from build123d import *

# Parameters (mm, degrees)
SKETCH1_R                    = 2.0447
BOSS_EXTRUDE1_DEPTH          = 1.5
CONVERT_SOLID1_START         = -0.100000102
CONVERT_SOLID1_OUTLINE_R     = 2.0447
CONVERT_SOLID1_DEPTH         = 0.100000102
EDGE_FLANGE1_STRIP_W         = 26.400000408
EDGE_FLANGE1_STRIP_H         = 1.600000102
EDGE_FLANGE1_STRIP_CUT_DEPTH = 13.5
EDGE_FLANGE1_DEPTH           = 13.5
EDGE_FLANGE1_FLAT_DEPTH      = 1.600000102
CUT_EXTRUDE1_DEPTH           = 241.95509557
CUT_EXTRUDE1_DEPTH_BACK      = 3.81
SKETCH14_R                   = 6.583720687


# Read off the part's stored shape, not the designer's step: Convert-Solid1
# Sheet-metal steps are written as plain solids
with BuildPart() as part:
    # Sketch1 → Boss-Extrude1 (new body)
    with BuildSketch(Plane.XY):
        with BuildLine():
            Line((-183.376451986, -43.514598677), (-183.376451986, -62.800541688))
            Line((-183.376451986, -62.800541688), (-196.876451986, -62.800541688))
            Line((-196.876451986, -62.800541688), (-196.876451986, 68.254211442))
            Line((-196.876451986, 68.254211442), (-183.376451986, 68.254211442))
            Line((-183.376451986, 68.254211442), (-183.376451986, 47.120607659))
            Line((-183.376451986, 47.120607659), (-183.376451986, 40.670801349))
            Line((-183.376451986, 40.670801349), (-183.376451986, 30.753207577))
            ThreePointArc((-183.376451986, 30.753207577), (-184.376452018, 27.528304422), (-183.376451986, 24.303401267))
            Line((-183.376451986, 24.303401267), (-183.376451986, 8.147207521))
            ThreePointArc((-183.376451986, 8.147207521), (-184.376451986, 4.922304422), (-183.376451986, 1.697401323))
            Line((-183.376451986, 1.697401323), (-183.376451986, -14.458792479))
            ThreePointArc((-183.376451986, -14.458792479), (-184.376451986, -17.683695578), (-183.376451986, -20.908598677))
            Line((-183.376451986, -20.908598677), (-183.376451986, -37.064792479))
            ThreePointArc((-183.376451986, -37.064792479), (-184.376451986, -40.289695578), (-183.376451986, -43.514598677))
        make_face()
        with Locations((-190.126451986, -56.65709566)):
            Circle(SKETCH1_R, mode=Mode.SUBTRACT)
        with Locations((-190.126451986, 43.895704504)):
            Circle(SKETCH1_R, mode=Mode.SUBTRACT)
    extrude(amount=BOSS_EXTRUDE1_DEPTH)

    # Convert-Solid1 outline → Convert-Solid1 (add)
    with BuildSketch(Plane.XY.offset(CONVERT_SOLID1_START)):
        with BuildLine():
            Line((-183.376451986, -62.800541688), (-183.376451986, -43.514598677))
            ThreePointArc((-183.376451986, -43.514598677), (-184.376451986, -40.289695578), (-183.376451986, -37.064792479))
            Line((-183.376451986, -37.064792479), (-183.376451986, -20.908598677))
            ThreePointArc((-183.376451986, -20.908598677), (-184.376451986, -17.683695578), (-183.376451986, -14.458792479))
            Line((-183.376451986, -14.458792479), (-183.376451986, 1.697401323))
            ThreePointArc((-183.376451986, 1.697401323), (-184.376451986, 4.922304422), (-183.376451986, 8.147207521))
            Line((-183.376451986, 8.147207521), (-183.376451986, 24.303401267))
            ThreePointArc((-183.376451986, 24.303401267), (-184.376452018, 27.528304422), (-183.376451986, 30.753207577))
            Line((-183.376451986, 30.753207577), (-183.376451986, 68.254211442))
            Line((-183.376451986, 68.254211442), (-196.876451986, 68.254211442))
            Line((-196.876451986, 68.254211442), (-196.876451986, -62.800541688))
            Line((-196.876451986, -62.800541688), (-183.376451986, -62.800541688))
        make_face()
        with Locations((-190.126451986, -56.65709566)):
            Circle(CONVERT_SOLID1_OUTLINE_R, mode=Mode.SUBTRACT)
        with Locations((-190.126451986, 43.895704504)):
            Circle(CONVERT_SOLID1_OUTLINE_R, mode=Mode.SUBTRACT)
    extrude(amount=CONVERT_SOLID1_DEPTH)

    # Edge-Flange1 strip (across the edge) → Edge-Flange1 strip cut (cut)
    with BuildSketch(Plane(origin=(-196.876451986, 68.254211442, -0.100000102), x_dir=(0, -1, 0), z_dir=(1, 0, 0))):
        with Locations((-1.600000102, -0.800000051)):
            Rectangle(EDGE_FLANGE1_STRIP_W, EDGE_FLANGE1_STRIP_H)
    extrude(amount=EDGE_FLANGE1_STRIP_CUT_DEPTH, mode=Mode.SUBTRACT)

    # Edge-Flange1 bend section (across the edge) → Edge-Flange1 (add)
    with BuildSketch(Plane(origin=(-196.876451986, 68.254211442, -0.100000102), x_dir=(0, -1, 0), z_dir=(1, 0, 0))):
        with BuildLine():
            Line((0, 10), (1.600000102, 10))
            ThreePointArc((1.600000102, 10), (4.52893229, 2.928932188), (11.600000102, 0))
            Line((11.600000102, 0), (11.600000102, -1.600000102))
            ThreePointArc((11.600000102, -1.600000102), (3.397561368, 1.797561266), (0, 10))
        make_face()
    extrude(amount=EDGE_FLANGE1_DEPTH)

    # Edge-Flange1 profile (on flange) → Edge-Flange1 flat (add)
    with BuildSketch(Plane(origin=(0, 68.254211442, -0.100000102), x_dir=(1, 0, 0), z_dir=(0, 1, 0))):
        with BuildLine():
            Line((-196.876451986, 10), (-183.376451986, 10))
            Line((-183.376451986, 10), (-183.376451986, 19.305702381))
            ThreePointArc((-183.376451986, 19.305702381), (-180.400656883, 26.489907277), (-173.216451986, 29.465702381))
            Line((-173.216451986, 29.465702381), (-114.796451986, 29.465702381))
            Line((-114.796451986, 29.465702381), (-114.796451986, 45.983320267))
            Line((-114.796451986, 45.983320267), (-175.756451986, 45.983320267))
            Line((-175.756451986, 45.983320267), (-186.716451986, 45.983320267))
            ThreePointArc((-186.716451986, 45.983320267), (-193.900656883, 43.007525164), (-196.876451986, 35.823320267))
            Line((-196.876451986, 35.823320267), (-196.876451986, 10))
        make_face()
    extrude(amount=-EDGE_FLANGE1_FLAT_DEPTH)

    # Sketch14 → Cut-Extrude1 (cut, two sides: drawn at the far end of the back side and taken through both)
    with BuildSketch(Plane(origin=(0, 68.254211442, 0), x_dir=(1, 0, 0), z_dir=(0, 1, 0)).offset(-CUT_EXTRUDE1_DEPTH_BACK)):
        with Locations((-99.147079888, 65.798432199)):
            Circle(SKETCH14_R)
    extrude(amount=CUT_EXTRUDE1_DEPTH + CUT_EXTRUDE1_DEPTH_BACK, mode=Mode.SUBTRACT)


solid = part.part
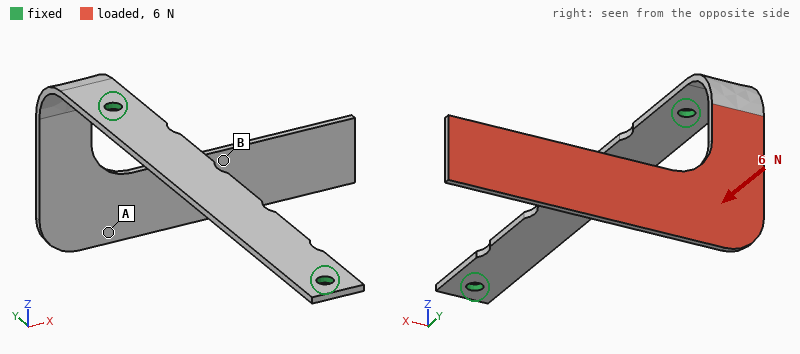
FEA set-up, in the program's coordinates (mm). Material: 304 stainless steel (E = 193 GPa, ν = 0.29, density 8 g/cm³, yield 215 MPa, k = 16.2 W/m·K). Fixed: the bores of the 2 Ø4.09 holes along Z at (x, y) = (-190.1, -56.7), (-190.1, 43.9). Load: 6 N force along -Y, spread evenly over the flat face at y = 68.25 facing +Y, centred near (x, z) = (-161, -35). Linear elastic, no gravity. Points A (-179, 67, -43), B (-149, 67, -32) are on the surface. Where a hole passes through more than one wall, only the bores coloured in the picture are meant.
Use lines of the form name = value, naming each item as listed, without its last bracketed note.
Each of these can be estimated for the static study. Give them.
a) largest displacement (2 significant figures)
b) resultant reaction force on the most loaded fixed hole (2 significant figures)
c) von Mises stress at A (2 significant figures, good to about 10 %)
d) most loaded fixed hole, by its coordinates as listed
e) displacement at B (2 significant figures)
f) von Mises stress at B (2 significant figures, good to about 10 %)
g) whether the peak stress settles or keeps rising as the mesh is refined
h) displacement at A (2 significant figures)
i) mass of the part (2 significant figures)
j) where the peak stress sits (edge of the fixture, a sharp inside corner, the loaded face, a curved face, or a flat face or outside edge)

largest displacement = 0.80 mm
resultant reaction force on the most loaded fixed hole = 6.0 N
von Mises stress at A = 14 MPa
most loaded fixed hole, by its coordinates as listed = (-190.1, 43.9)
displacement at B = 0.44 mm
von Mises stress at B = 5.2 MPa
whether the peak stress settles or keeps rising as the mesh is refined = keeps rising
displacement at A = 0.35 mm
mass of the part = 44 g
where the peak stress sits = edge of the fixture
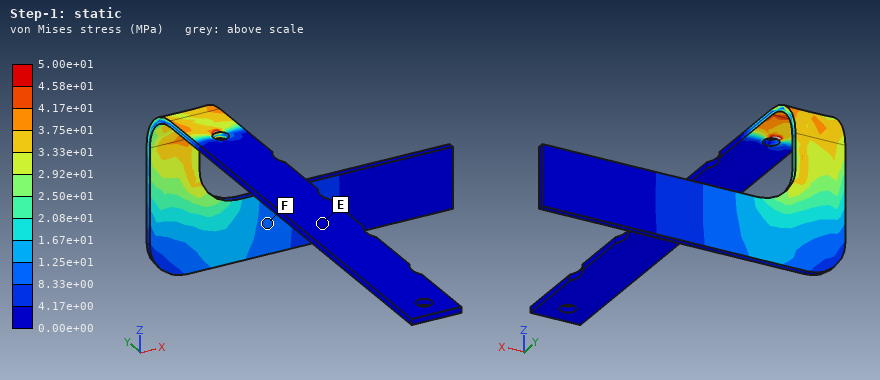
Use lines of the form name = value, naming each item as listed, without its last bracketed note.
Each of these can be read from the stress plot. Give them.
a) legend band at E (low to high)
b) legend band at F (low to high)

legend band at E = 0.00e+00 to 4.17e+00 MPa
legend band at F = 8.33e+00 to 1.25e+01 MPa
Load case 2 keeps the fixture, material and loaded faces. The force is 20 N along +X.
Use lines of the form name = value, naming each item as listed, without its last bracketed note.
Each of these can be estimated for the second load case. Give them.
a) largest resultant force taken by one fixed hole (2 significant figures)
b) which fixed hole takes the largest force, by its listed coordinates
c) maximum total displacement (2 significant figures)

largest resultant force taken by one fixed hole = 21 N
which fixed hole takes the largest force, by its listed coordinates = (-190.1, 43.9)
maximum total displacement = 0.85 mm
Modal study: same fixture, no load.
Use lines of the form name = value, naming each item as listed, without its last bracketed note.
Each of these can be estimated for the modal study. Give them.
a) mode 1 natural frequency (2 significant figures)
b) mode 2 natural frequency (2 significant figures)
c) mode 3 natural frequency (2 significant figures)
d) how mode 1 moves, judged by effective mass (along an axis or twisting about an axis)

mode 1 natural frequency = 120 Hz
mode 2 natural frequency = 180 Hz
mode 3 natural frequency = 320 Hz
how mode 1 moves, judged by effective mass = along Y
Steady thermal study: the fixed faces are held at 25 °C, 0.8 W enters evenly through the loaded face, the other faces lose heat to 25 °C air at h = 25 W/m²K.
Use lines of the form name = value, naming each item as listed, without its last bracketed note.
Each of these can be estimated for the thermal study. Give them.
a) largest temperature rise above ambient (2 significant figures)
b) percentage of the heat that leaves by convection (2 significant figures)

largest temperature rise above ambient = 15 K
percentage of the heat that leaves by convection = 93 %
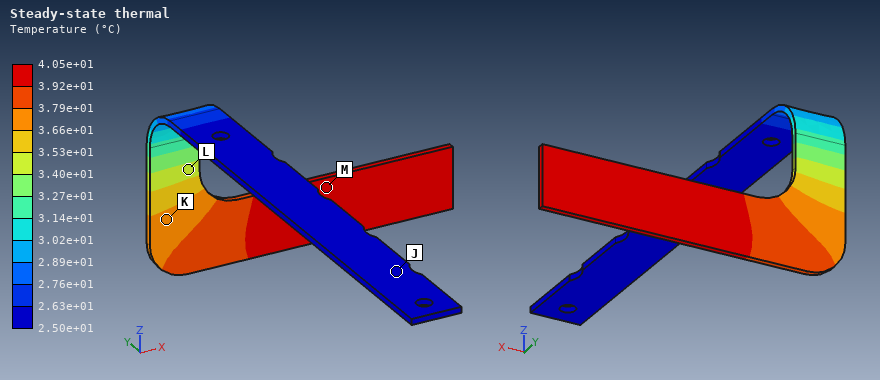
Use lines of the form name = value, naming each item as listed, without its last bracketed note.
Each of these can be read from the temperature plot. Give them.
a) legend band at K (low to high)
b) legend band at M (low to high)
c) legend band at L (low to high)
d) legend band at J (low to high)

legend band at K = 3.66e+01 to 3.79e+01 °C
legend band at M = 3.92e+01 to 4.05e+01 °C
legend band at L = 3.40e+01 to 3.53e+01 °C
legend band at J = 2.50e+01 to 2.63e+01 °C
